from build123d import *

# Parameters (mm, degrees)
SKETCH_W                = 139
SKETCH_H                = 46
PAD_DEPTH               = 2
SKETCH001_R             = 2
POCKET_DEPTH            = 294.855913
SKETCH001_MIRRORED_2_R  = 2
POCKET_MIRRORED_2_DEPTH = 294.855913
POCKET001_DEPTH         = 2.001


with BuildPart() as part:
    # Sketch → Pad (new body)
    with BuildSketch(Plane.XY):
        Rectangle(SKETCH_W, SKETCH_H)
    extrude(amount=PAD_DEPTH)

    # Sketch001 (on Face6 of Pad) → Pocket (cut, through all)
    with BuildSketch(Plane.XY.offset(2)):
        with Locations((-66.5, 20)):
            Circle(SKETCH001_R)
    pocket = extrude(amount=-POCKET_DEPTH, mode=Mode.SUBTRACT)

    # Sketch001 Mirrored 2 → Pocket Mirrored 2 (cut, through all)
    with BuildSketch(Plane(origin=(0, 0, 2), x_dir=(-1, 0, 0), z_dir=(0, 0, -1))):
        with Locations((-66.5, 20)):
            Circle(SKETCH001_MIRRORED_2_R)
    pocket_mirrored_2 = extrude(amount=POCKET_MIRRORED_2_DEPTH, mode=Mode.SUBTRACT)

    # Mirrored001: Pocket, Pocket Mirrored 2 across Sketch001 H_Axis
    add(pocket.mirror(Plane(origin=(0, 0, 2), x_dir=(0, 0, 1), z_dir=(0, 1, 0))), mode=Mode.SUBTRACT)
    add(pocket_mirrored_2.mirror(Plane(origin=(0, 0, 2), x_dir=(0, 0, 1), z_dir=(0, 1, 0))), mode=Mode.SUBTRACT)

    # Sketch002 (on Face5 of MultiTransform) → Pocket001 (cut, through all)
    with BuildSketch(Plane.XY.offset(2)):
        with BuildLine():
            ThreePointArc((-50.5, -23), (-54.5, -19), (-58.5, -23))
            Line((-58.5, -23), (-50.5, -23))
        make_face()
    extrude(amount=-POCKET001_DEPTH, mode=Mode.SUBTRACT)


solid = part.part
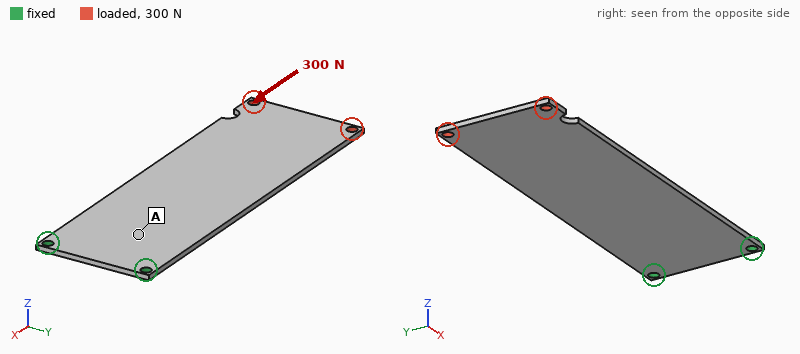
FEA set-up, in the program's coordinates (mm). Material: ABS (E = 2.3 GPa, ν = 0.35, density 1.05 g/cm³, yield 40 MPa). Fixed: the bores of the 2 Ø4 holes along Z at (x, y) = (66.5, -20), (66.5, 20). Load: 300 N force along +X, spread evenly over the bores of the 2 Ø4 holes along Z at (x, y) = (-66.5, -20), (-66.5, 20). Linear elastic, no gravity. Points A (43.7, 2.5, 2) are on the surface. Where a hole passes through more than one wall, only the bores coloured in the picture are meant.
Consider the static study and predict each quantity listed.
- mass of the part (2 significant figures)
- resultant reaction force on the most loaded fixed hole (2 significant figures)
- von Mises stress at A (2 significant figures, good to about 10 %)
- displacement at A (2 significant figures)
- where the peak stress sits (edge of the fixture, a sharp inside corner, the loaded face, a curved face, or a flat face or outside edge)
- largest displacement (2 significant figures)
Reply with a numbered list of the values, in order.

1. 13 g
2. 160 N
3. 2.3 MPa
4. 0.061 mm
5. the loaded face
6. 0.37 mm
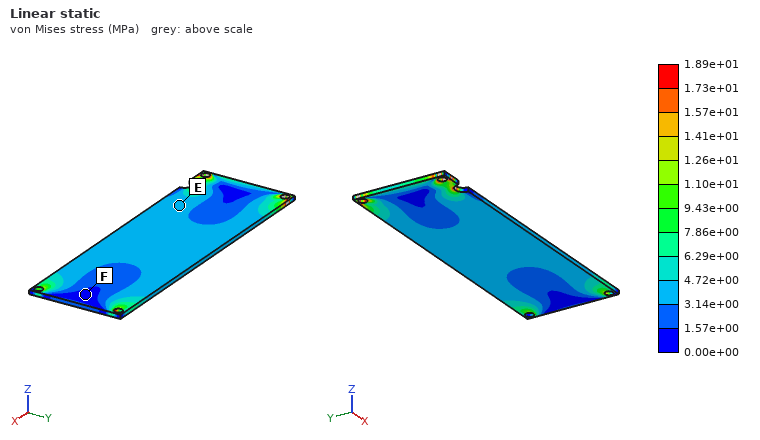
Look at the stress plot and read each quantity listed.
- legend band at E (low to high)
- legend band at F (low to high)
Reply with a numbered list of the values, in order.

1. 3.14e+00 to 4.72e+00 MPa
2. 0.00e+00 to 1.57e+00 MPa
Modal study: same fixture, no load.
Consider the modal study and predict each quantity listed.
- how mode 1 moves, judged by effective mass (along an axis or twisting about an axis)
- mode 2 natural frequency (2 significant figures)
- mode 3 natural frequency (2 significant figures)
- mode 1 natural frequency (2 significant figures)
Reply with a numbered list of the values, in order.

1. along Z
2. 160 Hz
3. 160 Hz
4. 25 Hz
